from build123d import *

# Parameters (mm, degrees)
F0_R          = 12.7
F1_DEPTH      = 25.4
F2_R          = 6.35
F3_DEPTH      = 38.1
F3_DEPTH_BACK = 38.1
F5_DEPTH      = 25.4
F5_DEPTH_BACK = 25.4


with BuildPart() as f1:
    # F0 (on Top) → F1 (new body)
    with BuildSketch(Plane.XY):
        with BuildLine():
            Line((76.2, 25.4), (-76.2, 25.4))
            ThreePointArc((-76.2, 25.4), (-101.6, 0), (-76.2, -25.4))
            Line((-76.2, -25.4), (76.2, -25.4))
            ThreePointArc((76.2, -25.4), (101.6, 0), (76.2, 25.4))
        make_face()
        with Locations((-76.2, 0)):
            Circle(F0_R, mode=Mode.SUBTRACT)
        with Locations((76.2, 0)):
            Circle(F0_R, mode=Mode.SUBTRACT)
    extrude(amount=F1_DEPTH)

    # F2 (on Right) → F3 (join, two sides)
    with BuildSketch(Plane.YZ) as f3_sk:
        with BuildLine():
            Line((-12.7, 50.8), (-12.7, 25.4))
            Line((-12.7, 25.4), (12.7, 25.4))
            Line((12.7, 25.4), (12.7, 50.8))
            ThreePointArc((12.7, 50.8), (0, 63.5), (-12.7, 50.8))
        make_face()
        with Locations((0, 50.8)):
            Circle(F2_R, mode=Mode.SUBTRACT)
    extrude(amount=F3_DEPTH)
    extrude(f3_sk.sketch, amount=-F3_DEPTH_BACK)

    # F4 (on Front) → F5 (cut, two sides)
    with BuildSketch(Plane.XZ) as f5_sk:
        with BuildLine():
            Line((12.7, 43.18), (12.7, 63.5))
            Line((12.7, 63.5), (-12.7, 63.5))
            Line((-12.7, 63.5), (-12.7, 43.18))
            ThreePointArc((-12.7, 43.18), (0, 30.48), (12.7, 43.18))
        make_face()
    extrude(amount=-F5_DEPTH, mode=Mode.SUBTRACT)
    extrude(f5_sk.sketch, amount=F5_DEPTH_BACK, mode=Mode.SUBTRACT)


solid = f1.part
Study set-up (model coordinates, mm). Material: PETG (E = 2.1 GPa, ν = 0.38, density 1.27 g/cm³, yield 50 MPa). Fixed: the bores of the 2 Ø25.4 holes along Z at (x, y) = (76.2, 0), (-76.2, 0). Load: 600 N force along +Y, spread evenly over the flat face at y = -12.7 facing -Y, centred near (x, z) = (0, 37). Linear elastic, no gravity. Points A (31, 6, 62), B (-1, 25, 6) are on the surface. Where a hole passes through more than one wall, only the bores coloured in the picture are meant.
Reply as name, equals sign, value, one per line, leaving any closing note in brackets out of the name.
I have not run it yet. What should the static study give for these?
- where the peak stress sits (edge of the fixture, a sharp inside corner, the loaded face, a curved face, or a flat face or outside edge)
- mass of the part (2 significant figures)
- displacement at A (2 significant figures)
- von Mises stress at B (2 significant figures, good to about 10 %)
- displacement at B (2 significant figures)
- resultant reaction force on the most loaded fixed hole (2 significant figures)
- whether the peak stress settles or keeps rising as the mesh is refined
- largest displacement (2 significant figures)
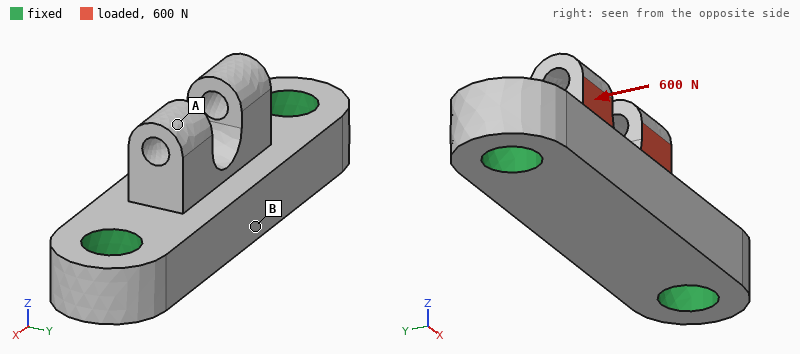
where the peak stress sits = edge of the fixture
mass of the part = 340 g
displacement at A = 0.13 mm
von Mises stress at B = 0.65 MPa
displacement at B = 0.048 mm
resultant reaction force on the most loaded fixed hole = 300 N
whether the peak stress settles or keeps rising as the mesh is refined = keeps rising
largest displacement = 0.14 mm
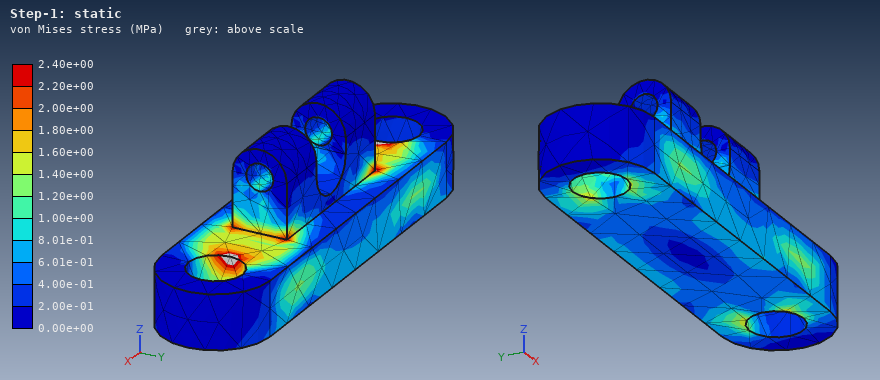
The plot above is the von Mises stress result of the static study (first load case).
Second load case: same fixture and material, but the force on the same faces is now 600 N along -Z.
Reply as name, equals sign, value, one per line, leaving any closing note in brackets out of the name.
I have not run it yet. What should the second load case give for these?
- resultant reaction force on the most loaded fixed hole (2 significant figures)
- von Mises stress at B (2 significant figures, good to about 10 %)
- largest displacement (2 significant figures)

resultant reaction force on the most loaded fixed hole = 310 N
von Mises stress at B = 0.30 MPa
largest displacement = 89 µm
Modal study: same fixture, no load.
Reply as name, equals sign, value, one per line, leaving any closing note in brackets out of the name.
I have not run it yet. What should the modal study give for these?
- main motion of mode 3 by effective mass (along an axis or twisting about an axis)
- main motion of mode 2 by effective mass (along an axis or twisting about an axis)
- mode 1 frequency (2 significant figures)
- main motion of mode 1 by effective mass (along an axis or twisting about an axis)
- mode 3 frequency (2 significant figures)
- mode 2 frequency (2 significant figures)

main motion of mode 3 by effective mass = along Y
main motion of mode 2 by effective mass = along Z
mode 1 frequency = 1300 Hz
main motion of mode 1 by effective mass = along Y
mode 3 frequency = 1900 Hz
mode 2 frequency = 1400 Hz
